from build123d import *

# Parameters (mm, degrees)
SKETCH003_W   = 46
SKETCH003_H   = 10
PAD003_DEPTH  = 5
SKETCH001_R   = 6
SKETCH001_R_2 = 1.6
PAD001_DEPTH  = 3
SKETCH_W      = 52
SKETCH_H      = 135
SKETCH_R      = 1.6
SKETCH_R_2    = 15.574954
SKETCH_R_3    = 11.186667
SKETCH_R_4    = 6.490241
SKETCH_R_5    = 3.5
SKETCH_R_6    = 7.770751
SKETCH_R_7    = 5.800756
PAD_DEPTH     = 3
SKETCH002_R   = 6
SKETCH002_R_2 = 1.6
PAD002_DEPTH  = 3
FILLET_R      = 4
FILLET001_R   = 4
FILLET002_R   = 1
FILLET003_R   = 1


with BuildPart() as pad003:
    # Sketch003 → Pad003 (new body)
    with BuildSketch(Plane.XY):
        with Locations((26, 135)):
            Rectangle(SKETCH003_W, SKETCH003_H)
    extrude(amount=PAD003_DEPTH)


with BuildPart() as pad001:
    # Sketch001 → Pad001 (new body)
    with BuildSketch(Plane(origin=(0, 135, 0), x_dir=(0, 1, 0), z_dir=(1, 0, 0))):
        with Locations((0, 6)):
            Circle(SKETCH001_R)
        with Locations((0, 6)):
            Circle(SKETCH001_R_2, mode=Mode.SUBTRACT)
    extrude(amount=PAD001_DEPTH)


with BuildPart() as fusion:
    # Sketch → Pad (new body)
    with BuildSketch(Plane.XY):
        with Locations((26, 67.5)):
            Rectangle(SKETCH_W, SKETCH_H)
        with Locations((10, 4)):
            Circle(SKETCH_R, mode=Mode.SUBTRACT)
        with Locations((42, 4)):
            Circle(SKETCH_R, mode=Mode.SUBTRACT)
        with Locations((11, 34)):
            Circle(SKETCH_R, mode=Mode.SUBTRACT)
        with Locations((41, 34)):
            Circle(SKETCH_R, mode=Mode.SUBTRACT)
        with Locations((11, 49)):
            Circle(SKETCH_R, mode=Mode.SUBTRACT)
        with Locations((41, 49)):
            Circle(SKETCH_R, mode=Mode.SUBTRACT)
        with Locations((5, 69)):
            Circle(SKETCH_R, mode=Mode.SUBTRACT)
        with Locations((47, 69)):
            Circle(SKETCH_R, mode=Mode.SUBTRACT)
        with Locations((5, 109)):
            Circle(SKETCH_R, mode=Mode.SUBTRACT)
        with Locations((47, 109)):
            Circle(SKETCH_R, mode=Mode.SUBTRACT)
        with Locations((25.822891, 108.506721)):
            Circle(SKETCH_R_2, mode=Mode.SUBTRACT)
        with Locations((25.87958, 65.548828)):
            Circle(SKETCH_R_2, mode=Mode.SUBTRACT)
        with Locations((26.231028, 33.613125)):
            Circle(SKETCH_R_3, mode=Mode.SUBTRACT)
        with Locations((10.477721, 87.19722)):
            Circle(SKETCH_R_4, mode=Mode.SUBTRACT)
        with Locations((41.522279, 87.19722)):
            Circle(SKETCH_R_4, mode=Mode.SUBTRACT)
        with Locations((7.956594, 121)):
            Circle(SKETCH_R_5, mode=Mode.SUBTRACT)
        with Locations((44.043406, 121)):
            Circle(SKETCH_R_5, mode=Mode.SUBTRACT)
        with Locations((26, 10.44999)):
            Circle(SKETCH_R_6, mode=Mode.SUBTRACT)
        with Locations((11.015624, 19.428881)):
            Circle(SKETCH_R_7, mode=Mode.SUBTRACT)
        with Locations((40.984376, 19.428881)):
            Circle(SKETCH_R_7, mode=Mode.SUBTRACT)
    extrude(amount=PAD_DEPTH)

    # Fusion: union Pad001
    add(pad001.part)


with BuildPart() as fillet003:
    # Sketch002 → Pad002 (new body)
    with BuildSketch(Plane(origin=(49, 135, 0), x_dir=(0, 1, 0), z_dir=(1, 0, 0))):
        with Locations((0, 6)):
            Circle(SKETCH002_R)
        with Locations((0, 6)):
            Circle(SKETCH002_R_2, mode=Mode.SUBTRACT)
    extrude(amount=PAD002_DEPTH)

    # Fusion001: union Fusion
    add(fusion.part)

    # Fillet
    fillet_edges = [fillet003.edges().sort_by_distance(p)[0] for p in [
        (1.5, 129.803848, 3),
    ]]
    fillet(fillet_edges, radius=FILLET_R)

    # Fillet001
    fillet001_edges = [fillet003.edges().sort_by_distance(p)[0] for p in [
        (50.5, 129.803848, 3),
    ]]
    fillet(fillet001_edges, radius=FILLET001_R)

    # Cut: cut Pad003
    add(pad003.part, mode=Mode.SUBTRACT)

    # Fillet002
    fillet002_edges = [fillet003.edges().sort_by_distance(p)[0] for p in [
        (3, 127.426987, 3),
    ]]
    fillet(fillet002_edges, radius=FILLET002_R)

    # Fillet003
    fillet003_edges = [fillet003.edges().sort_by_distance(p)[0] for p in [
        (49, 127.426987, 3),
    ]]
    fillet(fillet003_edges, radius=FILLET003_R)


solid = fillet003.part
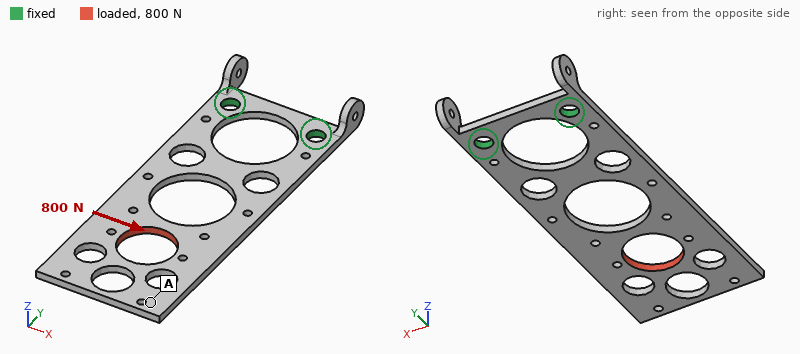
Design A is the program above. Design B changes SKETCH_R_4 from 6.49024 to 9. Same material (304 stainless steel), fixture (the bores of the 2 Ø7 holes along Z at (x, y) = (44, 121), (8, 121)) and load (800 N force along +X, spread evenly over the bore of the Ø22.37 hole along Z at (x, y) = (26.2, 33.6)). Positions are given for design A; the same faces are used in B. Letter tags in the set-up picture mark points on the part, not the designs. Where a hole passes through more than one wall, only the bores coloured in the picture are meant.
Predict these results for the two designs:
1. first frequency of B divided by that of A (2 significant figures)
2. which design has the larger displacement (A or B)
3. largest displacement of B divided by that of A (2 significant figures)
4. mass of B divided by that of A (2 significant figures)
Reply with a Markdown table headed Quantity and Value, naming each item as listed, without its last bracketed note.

| Quantity | Value |
|---|---|
| first frequency of B divided by that of A | 0.84 |
| which design has the larger displacement | B |
| largest displacement of B divided by that of A | 1.4 |
| mass of B divided by that of A | 0.94 |
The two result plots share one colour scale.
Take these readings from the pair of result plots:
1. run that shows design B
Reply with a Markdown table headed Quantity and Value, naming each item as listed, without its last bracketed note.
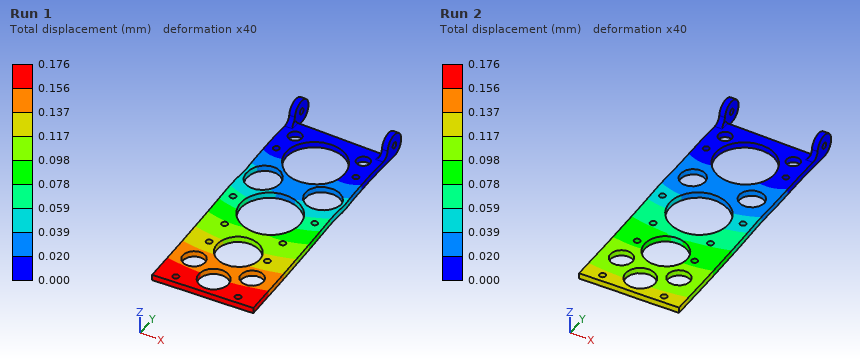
| Quantity | Value |
|---|---|
| run that shows design B | Run 1 |
